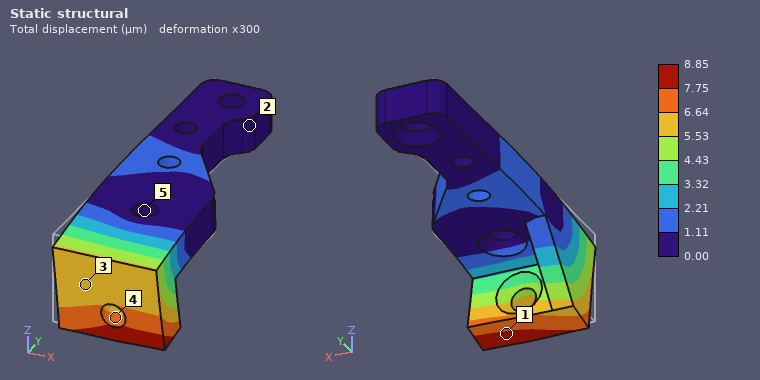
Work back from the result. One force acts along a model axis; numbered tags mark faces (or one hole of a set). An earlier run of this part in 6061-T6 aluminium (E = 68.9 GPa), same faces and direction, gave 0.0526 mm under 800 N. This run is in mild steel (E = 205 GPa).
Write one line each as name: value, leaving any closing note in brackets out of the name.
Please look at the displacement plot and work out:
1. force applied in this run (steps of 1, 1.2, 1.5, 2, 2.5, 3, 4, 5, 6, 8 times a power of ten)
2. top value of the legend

force applied in this run: 400 N
top value of the legend: 8.85 µm
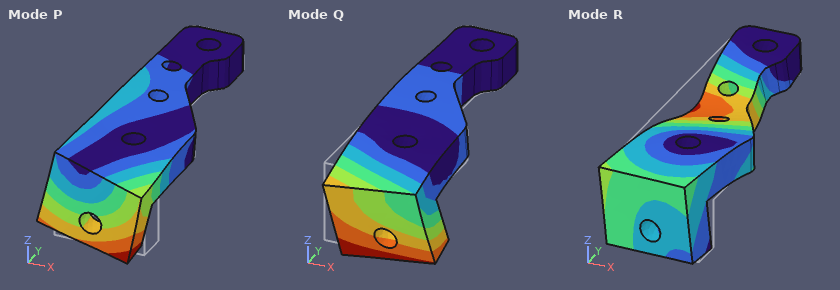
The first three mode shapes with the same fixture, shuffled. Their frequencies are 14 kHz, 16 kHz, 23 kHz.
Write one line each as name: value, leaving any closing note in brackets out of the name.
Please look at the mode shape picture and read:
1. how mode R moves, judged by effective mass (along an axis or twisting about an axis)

how mode R moves, judged by effective mass: along Z
